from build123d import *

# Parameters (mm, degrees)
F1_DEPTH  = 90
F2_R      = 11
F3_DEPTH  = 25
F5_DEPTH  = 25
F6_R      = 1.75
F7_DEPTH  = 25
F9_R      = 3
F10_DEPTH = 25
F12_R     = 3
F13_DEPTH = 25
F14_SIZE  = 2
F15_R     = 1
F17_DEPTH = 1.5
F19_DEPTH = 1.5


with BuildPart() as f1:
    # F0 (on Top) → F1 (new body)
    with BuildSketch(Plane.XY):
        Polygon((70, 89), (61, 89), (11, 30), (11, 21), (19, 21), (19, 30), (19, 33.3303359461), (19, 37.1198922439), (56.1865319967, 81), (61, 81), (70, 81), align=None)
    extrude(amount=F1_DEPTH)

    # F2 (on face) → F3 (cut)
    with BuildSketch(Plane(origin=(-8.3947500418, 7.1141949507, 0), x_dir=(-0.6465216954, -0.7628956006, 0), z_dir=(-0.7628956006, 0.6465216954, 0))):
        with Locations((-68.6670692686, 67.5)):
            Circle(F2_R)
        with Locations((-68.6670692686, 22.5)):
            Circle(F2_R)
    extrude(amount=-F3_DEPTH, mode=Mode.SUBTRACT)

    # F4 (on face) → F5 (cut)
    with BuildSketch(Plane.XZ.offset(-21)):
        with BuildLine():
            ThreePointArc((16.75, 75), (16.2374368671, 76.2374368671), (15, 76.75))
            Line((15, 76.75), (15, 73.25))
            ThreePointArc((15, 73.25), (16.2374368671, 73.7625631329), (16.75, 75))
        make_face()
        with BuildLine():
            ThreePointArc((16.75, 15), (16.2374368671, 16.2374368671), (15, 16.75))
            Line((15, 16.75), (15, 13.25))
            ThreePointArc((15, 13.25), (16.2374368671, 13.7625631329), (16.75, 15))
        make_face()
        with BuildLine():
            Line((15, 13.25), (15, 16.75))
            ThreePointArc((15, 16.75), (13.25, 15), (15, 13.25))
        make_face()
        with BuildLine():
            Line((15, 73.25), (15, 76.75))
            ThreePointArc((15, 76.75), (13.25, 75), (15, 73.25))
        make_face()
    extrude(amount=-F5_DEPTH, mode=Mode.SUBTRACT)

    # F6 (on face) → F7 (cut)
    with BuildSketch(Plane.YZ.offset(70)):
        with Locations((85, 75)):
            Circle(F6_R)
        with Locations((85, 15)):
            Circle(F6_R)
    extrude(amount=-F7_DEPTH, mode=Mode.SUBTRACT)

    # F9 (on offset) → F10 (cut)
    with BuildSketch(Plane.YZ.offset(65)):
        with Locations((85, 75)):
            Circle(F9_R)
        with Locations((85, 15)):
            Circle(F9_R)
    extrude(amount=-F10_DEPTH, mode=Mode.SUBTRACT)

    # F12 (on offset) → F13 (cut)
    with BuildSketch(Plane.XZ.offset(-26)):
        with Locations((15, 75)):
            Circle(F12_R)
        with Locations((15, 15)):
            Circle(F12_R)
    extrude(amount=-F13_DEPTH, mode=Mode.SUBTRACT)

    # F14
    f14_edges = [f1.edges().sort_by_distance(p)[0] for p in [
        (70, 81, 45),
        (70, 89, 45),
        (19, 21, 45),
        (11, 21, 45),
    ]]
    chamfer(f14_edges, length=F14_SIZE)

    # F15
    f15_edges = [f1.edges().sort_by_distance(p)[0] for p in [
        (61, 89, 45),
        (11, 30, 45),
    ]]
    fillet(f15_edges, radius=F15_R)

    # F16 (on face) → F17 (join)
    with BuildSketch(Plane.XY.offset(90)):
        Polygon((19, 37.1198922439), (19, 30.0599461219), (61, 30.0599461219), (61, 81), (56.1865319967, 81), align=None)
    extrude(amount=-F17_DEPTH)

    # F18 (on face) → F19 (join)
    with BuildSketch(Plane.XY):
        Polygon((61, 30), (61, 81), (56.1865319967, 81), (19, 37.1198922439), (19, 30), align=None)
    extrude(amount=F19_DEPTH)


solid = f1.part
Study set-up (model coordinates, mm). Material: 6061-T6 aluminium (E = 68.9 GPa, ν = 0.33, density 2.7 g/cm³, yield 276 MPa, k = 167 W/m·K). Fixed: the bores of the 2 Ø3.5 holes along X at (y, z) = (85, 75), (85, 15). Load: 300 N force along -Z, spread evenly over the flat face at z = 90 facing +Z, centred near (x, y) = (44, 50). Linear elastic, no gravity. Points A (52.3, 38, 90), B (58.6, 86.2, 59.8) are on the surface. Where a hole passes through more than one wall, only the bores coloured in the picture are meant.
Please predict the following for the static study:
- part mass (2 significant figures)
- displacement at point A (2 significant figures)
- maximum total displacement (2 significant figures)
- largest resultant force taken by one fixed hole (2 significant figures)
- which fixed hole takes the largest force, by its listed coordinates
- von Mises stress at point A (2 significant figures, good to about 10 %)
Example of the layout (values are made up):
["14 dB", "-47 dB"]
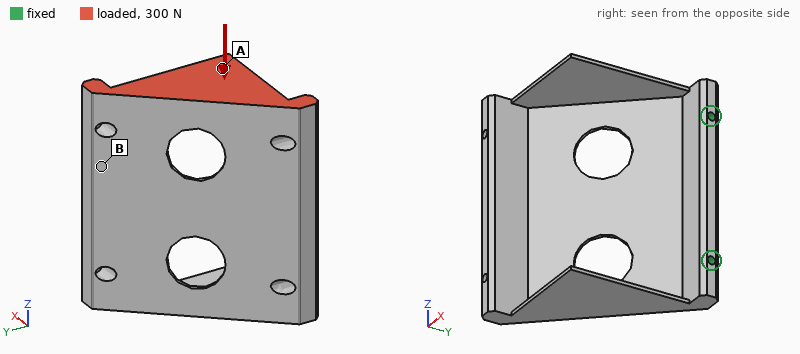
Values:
["74 g", "0.93 mm", "1.5 mm", "300 N", "(85, 75)", "33 MPa"]
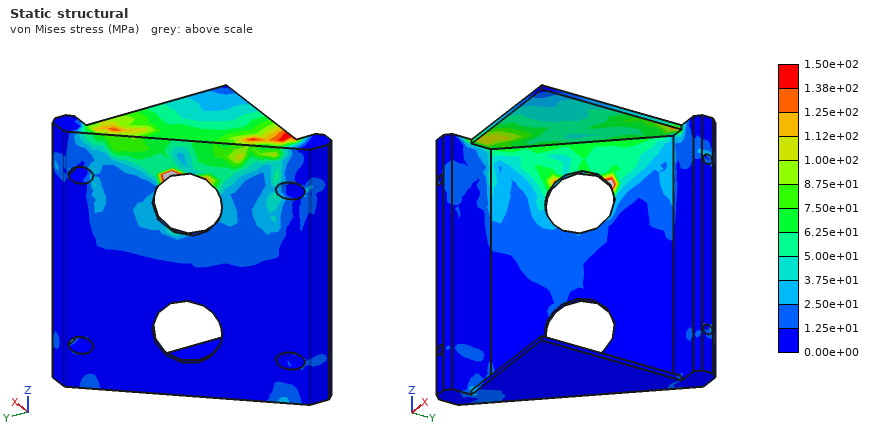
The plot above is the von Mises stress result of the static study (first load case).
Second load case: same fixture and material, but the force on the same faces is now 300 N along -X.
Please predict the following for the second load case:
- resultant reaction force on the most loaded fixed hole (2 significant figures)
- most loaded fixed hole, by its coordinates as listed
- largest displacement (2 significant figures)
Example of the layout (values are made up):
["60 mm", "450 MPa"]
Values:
["440 N", "(85, 75)", "1.4 mm"]
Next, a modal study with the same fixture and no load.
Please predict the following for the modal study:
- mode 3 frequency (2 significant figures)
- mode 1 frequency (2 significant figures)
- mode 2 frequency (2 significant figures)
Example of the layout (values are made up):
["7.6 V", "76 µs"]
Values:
["1300 Hz", "360 Hz", "740 Hz"]
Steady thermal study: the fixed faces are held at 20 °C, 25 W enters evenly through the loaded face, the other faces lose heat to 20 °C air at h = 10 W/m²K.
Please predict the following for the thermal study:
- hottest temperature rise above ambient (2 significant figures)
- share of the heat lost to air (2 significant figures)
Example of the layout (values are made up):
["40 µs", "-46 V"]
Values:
["71 K", "19 %"]
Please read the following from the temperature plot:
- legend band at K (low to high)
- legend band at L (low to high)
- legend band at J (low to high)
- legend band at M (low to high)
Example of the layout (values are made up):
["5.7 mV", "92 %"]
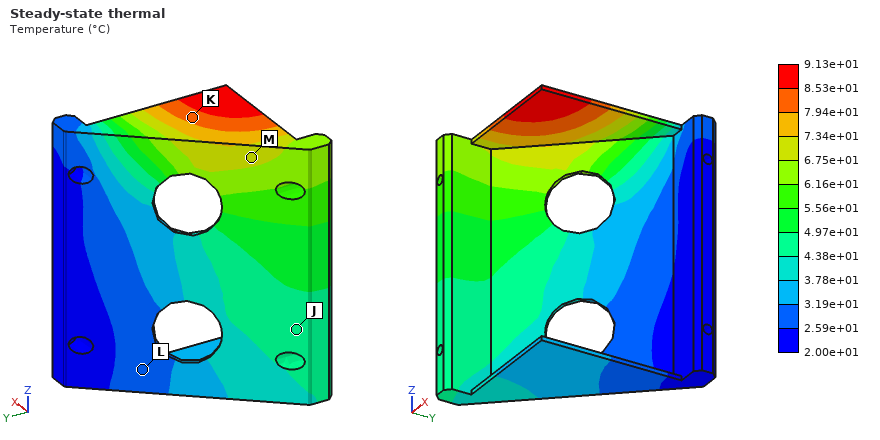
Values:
["7.94e+01 to 8.53e+01 °C", "2.59e+01 to 3.19e+01 °C", "4.38e+01 to 4.97e+01 °C", "6.75e+01 to 7.34e+01 °C"]
